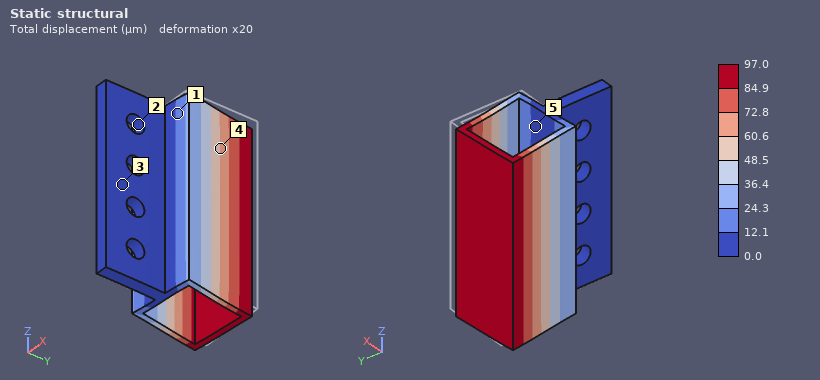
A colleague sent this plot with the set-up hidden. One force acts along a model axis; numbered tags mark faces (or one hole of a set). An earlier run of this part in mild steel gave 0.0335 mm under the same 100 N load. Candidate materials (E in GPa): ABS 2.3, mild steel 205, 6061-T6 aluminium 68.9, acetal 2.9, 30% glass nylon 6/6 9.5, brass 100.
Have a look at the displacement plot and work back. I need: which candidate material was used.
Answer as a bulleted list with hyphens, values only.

- 6061-T6 aluminium
